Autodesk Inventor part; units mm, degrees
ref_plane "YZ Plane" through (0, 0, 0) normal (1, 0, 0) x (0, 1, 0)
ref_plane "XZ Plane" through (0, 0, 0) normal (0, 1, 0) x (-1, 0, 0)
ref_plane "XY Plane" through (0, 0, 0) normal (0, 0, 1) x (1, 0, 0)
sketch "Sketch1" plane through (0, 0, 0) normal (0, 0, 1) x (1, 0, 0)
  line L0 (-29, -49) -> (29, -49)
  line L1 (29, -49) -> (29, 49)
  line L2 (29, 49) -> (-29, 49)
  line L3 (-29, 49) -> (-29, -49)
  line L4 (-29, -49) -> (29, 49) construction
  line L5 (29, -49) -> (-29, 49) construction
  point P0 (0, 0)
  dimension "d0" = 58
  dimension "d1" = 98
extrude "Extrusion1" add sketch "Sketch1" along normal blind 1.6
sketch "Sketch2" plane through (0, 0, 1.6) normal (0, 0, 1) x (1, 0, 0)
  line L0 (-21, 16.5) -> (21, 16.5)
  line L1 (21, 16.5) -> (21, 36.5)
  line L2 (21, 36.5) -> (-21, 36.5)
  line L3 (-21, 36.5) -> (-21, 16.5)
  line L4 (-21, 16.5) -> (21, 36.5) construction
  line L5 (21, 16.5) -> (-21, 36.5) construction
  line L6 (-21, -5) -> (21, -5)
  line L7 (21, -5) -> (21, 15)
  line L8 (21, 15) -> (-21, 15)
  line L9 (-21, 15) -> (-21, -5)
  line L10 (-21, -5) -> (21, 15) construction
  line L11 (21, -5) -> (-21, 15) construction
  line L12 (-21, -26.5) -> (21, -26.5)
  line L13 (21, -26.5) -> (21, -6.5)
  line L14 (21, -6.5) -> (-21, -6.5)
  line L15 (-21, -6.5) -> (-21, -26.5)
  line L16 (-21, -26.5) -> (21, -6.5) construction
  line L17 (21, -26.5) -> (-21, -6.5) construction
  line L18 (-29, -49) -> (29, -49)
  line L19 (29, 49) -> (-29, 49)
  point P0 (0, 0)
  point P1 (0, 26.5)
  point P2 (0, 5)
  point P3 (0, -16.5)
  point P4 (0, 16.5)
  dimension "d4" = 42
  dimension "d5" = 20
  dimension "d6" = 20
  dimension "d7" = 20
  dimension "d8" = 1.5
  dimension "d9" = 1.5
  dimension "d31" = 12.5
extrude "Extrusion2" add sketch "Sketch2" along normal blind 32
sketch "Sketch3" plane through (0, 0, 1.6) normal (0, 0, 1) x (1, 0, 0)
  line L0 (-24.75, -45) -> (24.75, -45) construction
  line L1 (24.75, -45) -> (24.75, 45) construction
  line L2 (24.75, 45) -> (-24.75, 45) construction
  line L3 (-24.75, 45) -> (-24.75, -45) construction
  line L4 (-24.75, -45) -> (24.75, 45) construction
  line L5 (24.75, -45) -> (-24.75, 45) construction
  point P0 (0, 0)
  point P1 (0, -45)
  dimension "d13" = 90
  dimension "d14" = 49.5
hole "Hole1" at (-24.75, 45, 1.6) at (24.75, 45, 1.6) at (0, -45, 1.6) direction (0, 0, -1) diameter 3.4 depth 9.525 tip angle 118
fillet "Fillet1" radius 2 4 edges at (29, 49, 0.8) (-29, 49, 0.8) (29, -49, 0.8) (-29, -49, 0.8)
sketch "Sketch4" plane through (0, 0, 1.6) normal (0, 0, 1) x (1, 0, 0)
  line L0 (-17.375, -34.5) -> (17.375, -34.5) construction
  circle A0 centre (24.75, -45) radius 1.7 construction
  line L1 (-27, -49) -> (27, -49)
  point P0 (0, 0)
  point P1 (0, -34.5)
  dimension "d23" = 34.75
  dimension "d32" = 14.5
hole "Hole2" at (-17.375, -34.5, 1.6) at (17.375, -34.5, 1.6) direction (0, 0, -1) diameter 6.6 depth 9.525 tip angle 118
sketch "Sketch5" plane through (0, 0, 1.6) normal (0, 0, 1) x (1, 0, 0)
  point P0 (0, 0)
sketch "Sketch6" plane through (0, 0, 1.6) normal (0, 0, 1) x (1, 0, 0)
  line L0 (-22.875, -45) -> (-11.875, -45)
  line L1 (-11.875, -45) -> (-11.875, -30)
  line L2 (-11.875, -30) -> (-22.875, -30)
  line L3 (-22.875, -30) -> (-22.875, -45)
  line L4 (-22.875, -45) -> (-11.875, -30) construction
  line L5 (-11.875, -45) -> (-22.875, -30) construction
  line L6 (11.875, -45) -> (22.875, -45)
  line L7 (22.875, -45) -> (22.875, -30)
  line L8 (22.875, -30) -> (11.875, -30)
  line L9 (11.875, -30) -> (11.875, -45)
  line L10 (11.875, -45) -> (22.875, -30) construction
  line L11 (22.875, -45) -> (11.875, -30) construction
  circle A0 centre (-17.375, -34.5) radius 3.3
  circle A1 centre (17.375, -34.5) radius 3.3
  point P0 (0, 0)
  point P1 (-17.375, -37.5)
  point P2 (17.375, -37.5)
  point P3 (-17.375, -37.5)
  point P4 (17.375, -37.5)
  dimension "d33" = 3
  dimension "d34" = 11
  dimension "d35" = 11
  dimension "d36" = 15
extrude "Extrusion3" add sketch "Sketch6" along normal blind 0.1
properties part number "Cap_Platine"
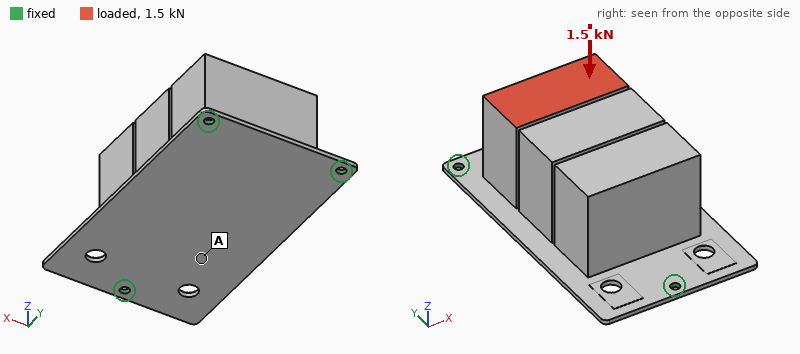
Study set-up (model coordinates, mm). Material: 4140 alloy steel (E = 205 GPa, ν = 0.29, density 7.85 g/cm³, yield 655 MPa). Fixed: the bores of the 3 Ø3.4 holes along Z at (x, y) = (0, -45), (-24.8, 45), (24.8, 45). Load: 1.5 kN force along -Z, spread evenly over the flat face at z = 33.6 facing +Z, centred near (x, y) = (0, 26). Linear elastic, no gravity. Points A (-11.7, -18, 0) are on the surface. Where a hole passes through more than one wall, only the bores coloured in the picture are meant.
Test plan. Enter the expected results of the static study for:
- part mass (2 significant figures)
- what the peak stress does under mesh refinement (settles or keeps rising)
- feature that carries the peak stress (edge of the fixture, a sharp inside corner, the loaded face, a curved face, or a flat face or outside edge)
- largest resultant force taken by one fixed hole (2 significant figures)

700 g
keeps rising
edge of the fixture
730 N
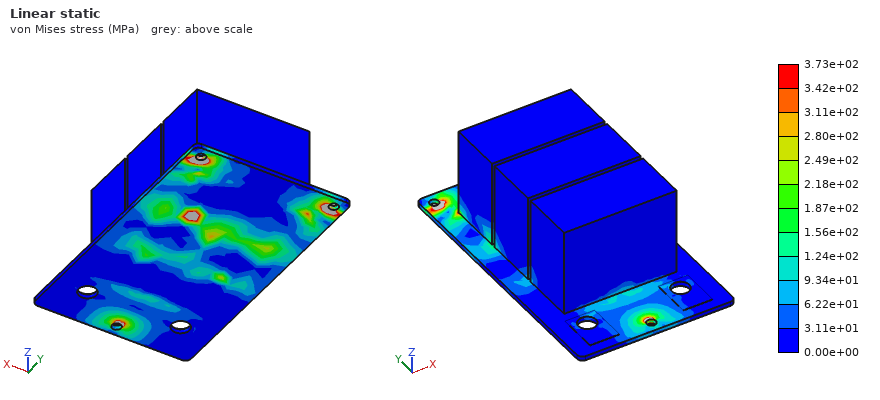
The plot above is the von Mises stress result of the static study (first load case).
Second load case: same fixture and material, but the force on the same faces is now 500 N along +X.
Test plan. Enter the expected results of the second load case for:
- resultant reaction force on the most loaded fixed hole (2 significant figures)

460 N
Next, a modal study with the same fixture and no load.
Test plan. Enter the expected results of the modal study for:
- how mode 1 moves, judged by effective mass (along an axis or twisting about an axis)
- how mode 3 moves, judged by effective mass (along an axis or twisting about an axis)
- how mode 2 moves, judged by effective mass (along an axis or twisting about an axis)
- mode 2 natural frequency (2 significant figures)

along Z
along Y
along X
820 Hz
